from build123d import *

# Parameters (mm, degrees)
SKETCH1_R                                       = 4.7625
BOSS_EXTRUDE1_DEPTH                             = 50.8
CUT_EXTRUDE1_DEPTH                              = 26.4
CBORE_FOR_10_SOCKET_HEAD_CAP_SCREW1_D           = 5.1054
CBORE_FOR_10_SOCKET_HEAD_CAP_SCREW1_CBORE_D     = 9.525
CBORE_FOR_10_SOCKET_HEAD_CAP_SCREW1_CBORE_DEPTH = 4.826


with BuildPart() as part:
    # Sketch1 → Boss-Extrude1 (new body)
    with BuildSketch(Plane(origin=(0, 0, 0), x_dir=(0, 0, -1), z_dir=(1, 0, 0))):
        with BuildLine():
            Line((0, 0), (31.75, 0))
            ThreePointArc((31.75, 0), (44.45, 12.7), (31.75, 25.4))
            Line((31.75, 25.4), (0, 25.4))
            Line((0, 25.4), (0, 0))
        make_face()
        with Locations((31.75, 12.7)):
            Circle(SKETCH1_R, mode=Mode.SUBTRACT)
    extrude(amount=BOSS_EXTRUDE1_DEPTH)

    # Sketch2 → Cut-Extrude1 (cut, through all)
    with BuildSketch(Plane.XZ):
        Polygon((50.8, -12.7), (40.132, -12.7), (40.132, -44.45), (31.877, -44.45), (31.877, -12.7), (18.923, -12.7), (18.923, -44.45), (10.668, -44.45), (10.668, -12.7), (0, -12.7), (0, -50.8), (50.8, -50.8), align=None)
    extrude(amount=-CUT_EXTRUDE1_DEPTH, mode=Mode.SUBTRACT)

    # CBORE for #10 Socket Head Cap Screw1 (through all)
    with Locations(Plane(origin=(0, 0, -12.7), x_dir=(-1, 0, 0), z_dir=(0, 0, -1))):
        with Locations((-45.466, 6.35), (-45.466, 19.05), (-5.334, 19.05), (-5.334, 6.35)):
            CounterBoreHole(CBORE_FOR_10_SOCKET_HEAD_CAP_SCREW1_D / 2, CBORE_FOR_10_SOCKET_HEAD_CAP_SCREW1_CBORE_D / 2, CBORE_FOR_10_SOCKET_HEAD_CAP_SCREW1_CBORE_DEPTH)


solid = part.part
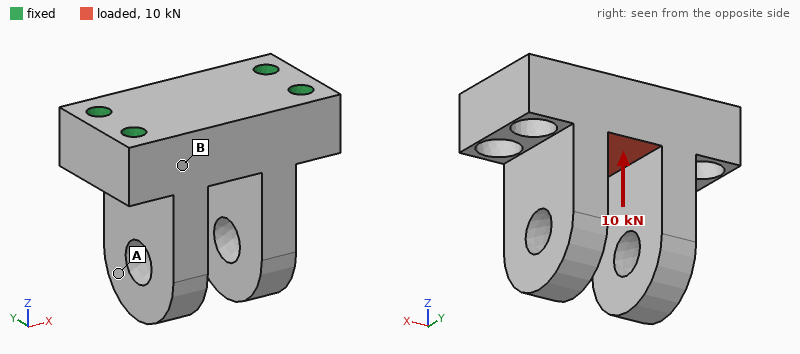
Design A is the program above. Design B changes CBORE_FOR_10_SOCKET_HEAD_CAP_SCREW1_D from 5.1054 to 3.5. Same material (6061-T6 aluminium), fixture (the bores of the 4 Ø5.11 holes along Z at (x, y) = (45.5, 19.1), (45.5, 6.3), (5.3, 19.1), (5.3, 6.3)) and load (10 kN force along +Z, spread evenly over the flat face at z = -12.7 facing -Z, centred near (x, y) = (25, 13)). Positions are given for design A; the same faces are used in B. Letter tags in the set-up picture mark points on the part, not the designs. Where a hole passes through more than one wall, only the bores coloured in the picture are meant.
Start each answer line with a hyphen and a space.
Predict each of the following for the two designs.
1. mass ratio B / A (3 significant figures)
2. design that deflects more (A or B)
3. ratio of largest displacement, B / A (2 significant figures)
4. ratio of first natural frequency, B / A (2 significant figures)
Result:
- 1.01
- B
- 1.1
- 0.99
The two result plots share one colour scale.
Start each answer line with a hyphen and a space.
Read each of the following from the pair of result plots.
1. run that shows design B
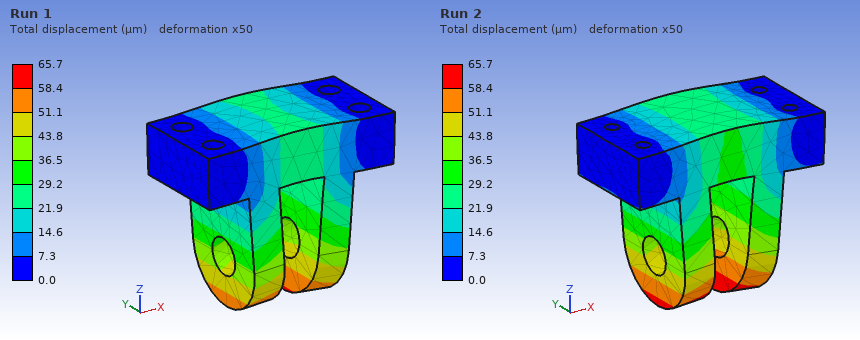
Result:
- Run 2
